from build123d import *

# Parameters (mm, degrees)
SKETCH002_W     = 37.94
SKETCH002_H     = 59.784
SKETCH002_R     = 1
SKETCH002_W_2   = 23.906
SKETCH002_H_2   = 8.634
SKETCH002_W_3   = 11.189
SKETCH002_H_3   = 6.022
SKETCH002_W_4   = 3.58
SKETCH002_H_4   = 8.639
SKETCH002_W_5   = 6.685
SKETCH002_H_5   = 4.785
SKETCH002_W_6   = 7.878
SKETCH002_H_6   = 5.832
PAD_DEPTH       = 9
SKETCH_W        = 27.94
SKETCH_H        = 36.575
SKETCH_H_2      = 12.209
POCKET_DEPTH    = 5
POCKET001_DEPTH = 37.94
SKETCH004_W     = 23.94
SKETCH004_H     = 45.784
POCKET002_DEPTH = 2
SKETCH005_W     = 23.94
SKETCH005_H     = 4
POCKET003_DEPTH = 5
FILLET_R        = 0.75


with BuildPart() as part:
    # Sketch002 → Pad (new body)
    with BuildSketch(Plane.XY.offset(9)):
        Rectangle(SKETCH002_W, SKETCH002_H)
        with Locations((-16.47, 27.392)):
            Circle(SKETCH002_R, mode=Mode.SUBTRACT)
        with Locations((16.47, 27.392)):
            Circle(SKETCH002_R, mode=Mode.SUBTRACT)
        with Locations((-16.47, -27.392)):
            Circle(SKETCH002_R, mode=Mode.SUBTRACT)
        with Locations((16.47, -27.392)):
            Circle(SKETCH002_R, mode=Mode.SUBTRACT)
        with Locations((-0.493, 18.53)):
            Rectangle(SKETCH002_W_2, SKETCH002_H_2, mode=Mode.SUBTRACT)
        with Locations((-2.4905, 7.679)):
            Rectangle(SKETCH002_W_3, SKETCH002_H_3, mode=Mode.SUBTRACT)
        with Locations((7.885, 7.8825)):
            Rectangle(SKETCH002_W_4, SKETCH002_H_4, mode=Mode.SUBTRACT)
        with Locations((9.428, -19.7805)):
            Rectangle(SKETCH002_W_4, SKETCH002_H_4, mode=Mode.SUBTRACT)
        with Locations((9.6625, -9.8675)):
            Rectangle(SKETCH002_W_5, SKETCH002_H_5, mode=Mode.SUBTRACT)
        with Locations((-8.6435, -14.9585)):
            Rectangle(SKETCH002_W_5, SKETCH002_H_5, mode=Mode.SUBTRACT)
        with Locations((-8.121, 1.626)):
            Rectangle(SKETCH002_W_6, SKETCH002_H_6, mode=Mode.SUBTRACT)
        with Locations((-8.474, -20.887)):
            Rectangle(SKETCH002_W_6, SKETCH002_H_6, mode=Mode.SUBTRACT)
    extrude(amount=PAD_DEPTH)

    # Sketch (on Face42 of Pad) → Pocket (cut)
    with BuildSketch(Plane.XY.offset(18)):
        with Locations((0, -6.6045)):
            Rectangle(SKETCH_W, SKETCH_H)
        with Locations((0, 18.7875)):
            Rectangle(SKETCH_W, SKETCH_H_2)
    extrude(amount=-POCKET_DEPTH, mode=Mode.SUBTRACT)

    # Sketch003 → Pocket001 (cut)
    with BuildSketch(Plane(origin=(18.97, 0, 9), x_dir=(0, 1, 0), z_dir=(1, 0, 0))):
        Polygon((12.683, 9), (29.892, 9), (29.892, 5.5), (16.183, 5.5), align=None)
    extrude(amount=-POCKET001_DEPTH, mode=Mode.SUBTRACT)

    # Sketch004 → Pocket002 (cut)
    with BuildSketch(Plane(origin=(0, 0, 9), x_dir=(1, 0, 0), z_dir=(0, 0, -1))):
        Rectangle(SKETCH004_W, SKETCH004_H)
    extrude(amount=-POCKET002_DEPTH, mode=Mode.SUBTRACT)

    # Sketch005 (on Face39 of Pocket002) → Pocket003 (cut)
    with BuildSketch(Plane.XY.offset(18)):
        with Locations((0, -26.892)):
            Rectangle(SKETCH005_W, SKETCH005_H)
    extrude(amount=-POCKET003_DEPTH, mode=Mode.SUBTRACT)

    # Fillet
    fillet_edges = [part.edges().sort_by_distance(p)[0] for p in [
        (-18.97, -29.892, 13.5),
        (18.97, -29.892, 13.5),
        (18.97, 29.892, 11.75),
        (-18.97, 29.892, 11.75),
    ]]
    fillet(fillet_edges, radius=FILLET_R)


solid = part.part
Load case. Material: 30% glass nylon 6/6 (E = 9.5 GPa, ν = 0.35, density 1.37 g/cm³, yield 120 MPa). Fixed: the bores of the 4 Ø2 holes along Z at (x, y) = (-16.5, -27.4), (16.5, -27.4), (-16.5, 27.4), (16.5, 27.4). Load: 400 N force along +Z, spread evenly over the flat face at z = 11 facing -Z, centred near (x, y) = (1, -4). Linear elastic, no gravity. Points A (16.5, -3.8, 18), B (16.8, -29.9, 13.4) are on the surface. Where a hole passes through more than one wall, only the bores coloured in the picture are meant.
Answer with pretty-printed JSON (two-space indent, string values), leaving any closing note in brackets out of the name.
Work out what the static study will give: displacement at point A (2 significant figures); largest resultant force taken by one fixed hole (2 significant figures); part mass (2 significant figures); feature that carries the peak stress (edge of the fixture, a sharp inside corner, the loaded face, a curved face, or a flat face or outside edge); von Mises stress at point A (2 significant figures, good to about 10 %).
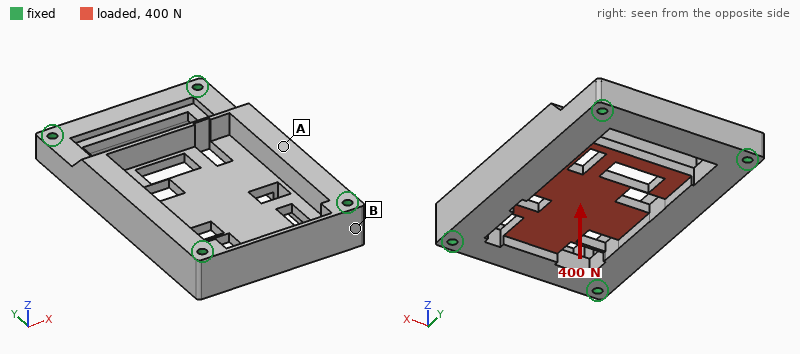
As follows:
{
  "displacement at point A": "0.076 mm",
  "largest resultant force taken by one fixed hole": "140 N",
  "part mass": "12 g",
  "feature that carries the peak stress": "a flat face or outside edge",
  "von Mises stress at point A": "11 MPa"
}
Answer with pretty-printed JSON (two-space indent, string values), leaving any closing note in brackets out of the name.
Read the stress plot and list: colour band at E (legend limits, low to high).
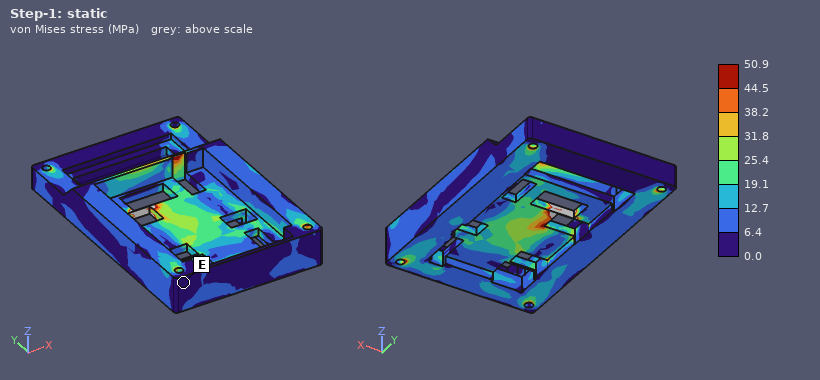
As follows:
{
  "colour band at E": "0.0 to 6.4 MPa"
}
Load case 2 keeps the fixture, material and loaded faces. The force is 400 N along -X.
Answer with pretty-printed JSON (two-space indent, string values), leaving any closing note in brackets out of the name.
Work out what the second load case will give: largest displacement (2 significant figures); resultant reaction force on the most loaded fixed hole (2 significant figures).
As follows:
{
  "largest displacement": "48 µm",
  "resultant reaction force on the most loaded fixed hole": "190 N"
}
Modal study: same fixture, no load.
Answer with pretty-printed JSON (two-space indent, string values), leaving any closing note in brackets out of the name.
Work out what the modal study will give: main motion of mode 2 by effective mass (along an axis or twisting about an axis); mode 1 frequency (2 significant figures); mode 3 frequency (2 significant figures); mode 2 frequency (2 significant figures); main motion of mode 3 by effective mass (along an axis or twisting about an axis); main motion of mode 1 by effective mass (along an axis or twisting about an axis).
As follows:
{
  "main motion of mode 2 by effective mass": "along X",
  "mode 1 frequency": "4500 Hz",
  "mode 3 frequency": "6400 Hz",
  "mode 2 frequency": "5600 Hz",
  "main motion of mode 3 by effective mass": "along X",
  "main motion of mode 1 by effective mass": "along Z"
}
